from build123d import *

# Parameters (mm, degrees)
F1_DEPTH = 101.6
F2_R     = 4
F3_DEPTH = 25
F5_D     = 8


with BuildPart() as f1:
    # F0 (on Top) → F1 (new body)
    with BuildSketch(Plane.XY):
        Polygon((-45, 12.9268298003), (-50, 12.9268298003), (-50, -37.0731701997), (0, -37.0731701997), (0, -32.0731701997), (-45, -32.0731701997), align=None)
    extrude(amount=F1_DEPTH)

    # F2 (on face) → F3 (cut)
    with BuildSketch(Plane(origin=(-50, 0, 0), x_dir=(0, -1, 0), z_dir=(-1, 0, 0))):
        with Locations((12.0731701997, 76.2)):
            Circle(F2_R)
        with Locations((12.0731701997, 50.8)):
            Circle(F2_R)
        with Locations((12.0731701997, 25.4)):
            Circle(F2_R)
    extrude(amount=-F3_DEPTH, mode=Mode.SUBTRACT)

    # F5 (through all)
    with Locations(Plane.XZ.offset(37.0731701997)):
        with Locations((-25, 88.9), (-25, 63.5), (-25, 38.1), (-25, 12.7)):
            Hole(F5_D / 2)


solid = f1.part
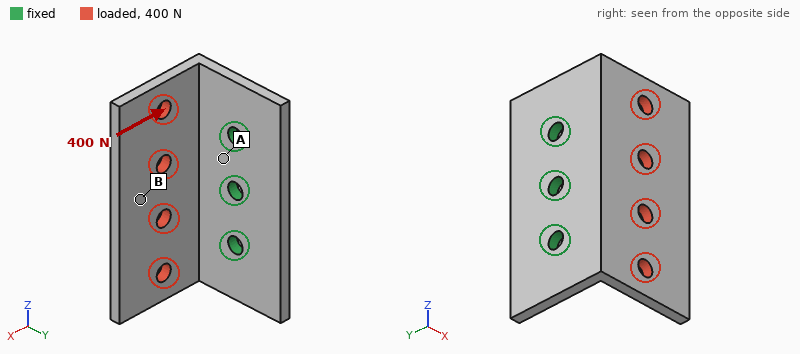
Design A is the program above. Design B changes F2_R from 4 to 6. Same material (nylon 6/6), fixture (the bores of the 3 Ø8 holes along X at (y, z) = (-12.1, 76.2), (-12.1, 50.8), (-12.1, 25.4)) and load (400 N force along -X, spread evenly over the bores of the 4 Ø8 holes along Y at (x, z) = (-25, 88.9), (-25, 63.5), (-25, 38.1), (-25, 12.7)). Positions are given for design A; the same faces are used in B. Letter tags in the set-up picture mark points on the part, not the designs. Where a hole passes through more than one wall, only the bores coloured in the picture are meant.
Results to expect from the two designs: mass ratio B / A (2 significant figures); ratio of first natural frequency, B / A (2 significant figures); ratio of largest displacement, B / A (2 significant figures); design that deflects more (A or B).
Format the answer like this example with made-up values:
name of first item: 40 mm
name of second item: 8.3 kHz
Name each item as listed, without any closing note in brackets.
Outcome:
mass ratio B / A: 0.98
ratio of first natural frequency, B / A: 1.1
ratio of largest displacement, B / A: 0.77
design that deflects more: A
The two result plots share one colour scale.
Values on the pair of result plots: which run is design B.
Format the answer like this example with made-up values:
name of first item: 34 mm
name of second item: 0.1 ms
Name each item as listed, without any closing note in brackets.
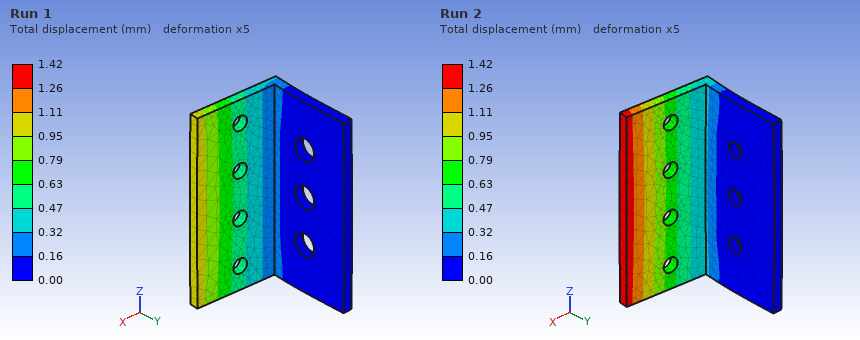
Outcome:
which run is design B: Run 1
